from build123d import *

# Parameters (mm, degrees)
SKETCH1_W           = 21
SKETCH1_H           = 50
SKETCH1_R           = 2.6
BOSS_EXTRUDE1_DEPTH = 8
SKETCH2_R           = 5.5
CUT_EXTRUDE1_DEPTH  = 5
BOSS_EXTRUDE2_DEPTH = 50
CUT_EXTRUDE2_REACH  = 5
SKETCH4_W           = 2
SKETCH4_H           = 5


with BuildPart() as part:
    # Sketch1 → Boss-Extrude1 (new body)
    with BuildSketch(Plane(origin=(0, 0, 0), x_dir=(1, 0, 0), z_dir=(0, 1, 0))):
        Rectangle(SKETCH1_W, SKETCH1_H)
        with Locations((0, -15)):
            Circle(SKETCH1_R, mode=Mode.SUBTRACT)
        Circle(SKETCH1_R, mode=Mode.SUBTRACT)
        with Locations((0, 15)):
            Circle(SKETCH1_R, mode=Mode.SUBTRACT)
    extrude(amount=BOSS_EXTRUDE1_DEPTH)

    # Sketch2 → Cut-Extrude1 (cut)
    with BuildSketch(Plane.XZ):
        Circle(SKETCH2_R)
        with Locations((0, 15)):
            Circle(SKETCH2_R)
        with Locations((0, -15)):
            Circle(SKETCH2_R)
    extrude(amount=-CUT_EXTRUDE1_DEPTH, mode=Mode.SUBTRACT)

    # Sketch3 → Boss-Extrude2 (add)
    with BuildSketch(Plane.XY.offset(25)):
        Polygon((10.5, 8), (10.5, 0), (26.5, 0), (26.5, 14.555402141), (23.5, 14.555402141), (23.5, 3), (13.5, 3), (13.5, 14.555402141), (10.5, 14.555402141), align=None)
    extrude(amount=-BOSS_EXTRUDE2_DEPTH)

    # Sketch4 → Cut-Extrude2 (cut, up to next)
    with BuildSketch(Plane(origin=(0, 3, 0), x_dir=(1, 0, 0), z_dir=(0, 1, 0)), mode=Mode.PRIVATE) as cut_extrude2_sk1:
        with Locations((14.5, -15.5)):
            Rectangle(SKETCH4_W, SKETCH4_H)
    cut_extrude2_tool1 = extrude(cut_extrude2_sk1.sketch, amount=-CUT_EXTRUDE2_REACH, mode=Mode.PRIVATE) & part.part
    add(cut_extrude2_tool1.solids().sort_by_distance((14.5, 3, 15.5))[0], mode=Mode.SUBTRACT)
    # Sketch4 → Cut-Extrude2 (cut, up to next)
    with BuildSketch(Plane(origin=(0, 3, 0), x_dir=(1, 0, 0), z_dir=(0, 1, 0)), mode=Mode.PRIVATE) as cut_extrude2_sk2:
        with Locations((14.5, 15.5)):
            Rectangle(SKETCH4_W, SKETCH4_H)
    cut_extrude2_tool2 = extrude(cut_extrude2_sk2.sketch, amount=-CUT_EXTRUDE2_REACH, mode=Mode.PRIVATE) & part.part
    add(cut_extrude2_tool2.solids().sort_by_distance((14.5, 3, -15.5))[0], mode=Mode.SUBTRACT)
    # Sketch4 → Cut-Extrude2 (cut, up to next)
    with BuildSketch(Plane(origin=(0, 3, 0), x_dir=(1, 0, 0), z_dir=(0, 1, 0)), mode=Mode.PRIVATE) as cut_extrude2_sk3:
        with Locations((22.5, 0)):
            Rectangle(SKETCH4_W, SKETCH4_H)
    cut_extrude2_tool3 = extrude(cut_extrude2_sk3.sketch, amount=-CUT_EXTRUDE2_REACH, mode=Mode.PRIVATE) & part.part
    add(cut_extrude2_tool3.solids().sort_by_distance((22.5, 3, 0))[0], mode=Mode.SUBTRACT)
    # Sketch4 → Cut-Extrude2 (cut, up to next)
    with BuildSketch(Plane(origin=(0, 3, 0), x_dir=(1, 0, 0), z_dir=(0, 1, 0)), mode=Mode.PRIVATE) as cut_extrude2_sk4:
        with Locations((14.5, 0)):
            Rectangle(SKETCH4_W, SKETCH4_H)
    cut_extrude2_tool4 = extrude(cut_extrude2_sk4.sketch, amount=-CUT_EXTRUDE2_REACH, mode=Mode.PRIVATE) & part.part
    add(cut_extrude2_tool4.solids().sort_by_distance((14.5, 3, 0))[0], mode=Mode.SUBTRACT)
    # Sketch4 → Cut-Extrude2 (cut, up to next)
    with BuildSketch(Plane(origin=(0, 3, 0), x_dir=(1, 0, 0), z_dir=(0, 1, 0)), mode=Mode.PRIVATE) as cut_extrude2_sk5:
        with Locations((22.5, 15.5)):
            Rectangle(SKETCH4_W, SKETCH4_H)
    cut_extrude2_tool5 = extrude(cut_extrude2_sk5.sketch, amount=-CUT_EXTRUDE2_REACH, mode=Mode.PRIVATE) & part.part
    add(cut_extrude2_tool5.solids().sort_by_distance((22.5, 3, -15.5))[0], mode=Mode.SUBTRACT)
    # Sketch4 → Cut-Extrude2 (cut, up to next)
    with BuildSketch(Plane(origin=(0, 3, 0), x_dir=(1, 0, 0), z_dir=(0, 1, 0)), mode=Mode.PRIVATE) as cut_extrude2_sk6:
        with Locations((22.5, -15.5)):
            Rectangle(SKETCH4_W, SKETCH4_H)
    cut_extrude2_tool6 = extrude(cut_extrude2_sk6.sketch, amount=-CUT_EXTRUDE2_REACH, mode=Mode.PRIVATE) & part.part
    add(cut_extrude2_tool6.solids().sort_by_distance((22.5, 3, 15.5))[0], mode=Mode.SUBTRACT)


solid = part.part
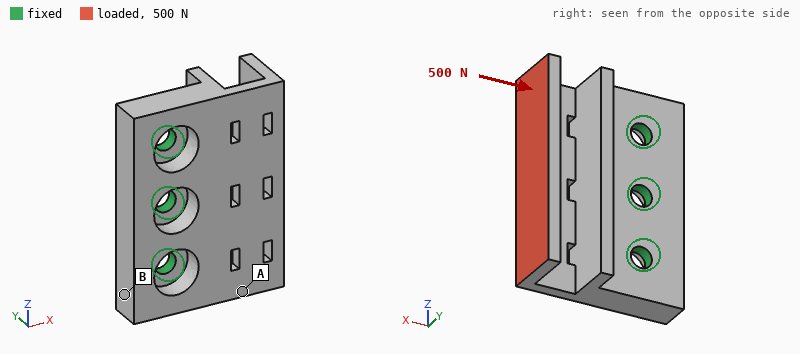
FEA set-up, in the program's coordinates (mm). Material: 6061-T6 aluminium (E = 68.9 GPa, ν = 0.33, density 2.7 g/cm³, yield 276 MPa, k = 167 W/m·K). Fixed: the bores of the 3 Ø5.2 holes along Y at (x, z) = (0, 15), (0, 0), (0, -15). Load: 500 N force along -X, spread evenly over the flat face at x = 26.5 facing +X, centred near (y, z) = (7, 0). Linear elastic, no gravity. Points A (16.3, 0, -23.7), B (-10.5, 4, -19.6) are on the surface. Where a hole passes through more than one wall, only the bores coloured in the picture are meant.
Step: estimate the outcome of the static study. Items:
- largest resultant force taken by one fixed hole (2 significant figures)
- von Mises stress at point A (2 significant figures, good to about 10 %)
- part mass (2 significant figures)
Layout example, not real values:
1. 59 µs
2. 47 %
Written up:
1. 180 N
2. 45 MPa
3. 34 g
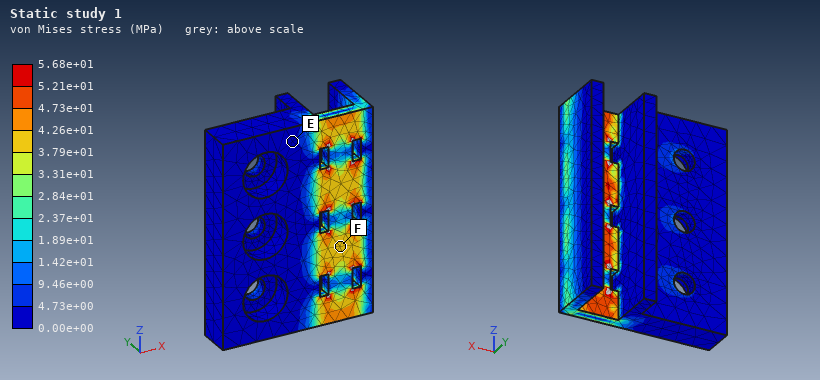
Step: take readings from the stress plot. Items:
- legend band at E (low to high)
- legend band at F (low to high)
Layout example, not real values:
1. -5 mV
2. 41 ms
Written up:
1. 0.00e+00 to 4.73e+00 MPa
2. 3.79e+01 to 4.26e+01 MPa
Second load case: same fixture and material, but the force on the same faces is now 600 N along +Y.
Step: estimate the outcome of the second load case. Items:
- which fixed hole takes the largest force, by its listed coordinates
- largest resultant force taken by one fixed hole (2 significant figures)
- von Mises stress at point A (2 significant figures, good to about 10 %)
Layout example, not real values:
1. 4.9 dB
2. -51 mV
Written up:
1. (0, 0)
2. 240 N
3. 110 MPa
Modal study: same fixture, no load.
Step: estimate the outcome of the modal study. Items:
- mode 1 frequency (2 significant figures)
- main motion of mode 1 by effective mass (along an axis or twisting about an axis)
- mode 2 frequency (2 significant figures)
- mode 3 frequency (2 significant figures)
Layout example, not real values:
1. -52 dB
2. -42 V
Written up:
1. 3500 Hz
2. along Y
3. 5500 Hz
4. 7400 Hz
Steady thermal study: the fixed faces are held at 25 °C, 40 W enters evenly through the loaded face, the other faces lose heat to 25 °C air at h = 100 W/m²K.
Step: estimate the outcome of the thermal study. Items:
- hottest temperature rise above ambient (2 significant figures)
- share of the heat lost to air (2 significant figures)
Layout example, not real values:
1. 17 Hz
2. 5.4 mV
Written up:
1. 40 K
2. 20 %
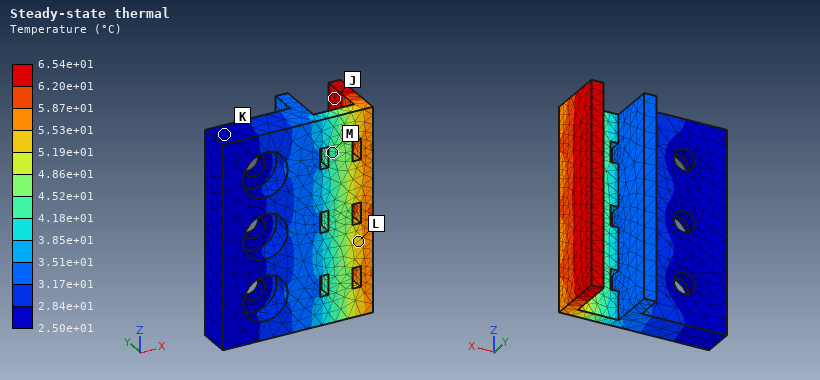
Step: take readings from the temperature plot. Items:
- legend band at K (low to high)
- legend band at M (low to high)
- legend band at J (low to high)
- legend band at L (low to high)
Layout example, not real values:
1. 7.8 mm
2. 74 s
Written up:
1. 2.50e+01 to 2.84e+01 °C
2. 4.18e+01 to 4.52e+01 °C
3. 6.20e+01 to 6.54e+01 °C
4. 5.19e+01 to 5.53e+01 °C
